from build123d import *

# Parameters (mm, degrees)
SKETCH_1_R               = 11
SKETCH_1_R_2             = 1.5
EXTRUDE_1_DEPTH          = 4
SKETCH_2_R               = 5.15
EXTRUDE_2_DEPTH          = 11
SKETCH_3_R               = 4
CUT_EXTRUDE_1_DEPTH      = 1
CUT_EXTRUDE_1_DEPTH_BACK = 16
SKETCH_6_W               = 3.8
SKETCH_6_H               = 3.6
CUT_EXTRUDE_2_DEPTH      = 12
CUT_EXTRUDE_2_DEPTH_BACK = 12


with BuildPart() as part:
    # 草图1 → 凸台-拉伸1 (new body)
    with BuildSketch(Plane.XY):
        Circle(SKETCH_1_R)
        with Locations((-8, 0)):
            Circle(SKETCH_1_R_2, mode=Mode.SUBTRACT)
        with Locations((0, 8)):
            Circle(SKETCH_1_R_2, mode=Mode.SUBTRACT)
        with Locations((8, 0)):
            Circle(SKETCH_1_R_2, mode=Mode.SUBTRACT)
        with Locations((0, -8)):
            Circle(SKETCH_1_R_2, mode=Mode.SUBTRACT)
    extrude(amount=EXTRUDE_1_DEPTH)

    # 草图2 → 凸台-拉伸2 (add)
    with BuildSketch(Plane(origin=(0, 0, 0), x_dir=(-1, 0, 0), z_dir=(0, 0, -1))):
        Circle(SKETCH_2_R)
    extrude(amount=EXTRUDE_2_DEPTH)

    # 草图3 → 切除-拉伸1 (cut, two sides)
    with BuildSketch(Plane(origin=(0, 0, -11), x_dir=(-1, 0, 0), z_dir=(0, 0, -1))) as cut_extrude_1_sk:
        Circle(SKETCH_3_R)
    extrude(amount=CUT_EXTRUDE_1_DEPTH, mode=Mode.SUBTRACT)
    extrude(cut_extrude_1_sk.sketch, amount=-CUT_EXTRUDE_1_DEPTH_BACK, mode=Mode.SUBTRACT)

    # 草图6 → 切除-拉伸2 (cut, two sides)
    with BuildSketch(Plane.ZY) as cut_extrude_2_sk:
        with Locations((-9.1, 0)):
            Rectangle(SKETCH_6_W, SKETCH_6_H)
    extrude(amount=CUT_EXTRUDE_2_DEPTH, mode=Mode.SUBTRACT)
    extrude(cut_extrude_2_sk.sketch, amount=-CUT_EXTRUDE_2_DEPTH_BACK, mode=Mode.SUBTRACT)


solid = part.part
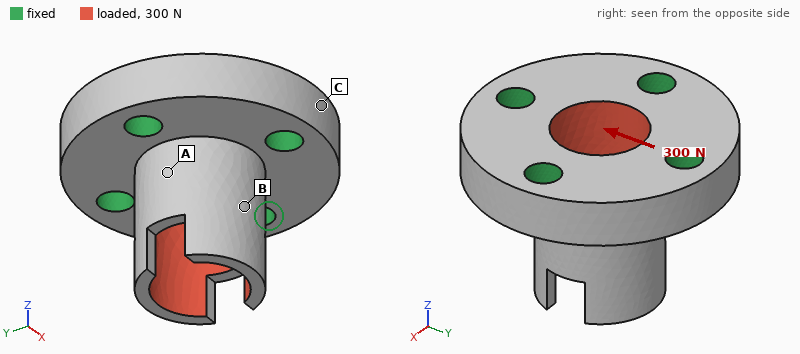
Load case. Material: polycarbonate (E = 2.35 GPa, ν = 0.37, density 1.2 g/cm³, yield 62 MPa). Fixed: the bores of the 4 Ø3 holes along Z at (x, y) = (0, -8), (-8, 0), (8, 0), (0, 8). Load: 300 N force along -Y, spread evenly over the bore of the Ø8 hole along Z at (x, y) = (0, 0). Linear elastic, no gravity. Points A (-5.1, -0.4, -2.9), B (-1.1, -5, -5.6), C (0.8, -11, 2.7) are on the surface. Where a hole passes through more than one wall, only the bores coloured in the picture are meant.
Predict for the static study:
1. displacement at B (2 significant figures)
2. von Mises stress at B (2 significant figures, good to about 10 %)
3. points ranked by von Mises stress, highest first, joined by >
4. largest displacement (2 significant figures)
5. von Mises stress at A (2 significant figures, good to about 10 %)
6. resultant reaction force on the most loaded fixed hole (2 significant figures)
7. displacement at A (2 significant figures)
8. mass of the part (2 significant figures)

0.12 mm
8.4 MPa
A > B > C
0.22 mm
15 MPa
140 N
0.056 mm
1.8 g
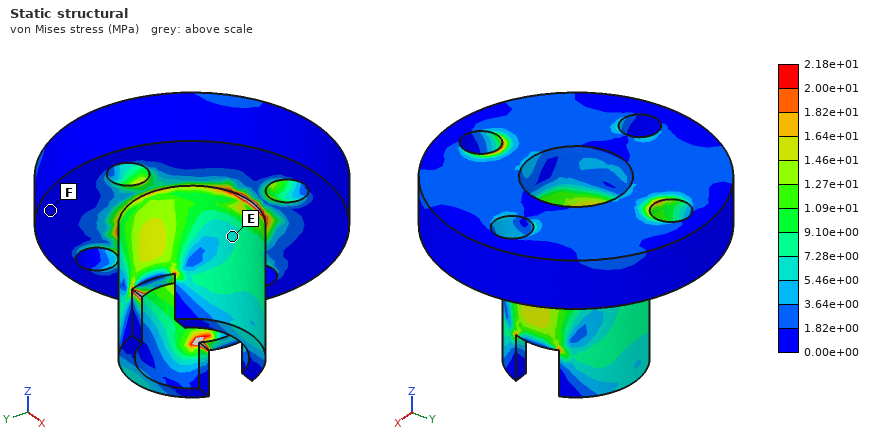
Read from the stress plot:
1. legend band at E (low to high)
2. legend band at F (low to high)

5.46e+00 to 7.28e+00 MPa
0.00e+00 to 1.82e+00 MPa
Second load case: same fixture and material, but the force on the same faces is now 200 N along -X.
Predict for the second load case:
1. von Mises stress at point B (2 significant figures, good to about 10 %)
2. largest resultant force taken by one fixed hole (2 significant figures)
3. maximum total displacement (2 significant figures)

4.4 MPa
91 N
0.17 mm
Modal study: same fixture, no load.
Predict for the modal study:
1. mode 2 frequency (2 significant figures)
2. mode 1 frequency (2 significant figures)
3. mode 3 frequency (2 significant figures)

9700 Hz
8600 Hz
9700 Hz
